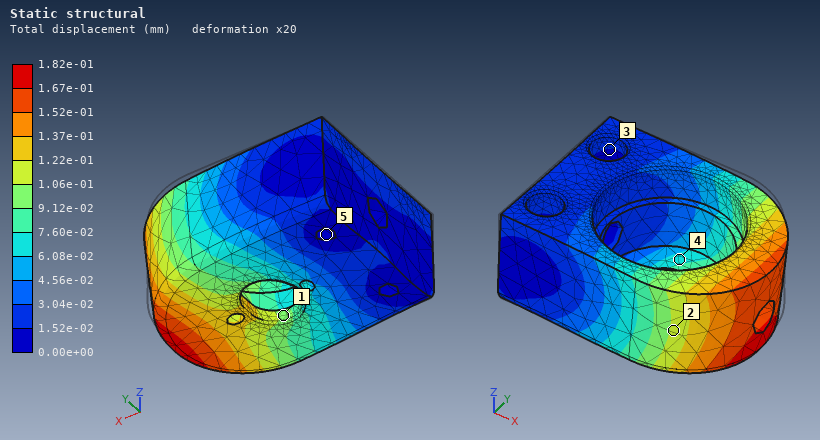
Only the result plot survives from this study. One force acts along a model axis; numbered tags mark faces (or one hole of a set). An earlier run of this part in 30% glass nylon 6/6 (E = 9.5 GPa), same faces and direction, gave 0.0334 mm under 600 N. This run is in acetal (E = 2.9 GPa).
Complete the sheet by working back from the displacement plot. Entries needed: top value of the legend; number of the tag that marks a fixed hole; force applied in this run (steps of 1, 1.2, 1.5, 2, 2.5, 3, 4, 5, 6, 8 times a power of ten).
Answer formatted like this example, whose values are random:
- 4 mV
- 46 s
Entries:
- 1.82e-01 mm
- 5
- 1 kN
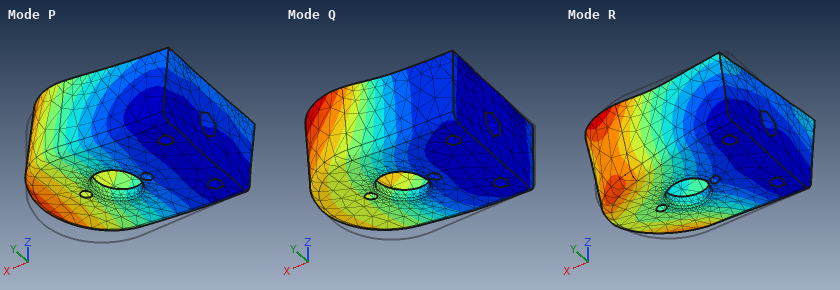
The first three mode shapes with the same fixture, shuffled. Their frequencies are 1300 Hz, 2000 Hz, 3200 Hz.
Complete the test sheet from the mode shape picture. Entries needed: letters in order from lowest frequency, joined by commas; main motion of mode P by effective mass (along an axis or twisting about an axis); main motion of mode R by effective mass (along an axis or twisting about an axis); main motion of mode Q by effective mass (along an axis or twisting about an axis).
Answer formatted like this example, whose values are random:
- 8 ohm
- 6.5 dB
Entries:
- P, Q, R
- along Z
- twisting about X
- along Y
